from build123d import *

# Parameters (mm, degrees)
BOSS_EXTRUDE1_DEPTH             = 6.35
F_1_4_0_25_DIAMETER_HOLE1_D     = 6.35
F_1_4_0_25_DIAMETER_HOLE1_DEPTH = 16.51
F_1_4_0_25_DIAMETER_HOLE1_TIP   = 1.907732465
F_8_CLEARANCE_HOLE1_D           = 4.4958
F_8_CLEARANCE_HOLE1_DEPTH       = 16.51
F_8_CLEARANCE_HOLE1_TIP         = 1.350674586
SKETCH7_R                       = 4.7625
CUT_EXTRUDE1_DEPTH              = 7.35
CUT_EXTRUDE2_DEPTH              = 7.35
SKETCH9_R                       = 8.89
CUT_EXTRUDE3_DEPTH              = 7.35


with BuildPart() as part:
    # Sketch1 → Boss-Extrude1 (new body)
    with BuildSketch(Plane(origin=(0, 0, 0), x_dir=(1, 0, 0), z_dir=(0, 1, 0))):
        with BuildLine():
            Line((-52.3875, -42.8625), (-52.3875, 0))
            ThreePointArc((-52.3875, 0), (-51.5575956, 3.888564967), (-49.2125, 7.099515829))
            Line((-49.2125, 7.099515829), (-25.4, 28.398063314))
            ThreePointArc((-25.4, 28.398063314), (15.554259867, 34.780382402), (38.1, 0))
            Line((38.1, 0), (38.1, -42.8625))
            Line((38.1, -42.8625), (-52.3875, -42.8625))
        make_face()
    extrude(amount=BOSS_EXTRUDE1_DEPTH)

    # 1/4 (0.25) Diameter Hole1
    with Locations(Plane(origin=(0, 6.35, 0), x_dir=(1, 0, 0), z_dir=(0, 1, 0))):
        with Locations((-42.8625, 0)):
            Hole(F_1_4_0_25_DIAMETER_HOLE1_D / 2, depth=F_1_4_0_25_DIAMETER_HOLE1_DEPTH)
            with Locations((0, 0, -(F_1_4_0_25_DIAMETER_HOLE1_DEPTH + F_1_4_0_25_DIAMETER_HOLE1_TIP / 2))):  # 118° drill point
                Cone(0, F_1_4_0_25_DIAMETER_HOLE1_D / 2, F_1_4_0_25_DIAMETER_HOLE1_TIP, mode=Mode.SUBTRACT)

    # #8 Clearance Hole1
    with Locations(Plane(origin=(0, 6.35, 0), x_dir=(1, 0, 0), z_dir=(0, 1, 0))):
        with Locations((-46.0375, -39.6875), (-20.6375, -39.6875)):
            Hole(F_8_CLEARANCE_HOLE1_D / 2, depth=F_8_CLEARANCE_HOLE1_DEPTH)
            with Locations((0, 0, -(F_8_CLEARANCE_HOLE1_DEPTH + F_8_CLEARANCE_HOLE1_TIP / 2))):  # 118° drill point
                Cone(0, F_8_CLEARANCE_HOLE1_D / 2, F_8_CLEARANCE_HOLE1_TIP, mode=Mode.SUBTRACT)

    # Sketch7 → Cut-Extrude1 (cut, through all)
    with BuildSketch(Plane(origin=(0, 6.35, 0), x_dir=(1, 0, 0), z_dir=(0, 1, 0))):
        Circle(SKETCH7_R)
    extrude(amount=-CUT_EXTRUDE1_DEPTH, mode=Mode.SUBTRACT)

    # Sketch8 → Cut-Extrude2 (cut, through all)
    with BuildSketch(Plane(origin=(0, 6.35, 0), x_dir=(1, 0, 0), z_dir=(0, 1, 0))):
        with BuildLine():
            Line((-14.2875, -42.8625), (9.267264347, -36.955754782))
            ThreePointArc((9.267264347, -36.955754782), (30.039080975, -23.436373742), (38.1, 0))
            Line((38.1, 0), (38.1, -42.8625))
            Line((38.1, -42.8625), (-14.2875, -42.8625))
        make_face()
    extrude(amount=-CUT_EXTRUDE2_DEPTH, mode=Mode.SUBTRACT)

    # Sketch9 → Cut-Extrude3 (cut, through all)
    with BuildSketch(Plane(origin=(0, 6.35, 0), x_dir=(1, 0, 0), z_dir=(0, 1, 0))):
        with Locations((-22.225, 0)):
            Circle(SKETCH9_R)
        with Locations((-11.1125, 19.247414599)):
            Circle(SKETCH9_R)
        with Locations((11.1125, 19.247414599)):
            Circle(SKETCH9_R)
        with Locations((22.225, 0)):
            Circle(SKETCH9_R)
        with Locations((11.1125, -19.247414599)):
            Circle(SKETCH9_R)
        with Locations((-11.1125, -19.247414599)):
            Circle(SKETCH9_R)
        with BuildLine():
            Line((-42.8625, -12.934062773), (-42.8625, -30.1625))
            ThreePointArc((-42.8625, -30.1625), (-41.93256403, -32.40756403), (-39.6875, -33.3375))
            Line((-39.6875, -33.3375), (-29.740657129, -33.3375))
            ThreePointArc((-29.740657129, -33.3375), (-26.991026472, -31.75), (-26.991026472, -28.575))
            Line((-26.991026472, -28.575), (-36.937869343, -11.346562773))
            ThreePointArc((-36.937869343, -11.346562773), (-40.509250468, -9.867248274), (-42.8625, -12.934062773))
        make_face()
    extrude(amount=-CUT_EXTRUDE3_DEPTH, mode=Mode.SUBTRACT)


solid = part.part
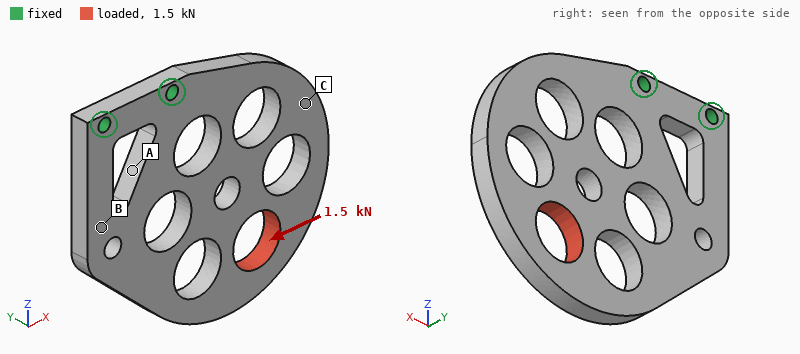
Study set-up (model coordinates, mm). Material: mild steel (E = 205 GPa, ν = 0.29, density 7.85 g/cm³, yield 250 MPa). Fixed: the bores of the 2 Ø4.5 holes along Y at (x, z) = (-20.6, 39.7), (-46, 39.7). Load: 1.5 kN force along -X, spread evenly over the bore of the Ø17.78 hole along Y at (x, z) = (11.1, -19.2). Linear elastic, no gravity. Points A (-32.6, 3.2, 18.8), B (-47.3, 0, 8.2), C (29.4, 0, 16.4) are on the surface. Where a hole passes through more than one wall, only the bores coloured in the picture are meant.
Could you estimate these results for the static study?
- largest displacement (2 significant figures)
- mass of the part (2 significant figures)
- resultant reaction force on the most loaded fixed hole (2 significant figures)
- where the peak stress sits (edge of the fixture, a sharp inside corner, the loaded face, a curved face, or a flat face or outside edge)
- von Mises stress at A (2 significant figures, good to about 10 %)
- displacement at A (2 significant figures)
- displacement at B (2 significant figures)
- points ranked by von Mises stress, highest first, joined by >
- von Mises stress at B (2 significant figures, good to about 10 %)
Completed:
60 µm
200 g
2.9 kN
edge of the fixture
49 MPa
14 µm
21 µm
A > B > C
26 MPa
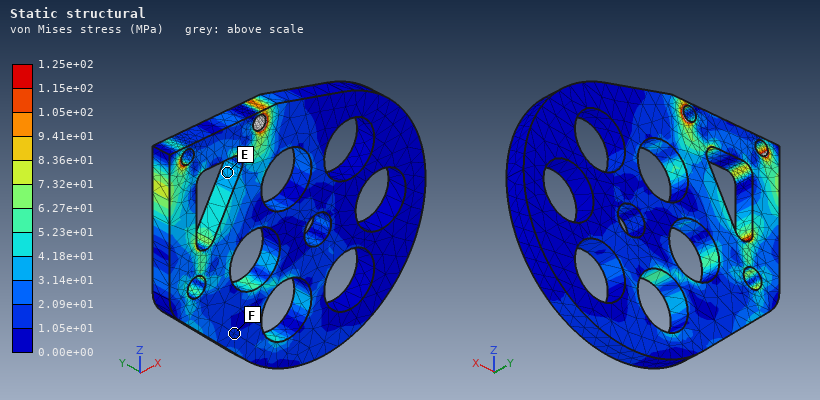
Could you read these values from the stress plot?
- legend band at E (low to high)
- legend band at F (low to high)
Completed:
3.14e+01 to 4.18e+01 MPa
1.05e+01 to 2.09e+01 MPa
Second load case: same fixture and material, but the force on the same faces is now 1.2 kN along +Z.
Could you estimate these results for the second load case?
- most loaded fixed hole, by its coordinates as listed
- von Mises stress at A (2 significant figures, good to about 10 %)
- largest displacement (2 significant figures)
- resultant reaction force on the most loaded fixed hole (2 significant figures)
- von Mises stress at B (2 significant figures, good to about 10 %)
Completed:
(-20.6, 39.7)
18 MPa
35 µm
2.3 kN
11 MPa
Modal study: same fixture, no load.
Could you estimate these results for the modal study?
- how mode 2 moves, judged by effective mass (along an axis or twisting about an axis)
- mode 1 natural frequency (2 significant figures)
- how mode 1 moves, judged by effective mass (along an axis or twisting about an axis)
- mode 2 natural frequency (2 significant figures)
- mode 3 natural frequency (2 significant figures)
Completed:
twisting about Z
630 Hz
along Y
1400 Hz
2500 Hz
